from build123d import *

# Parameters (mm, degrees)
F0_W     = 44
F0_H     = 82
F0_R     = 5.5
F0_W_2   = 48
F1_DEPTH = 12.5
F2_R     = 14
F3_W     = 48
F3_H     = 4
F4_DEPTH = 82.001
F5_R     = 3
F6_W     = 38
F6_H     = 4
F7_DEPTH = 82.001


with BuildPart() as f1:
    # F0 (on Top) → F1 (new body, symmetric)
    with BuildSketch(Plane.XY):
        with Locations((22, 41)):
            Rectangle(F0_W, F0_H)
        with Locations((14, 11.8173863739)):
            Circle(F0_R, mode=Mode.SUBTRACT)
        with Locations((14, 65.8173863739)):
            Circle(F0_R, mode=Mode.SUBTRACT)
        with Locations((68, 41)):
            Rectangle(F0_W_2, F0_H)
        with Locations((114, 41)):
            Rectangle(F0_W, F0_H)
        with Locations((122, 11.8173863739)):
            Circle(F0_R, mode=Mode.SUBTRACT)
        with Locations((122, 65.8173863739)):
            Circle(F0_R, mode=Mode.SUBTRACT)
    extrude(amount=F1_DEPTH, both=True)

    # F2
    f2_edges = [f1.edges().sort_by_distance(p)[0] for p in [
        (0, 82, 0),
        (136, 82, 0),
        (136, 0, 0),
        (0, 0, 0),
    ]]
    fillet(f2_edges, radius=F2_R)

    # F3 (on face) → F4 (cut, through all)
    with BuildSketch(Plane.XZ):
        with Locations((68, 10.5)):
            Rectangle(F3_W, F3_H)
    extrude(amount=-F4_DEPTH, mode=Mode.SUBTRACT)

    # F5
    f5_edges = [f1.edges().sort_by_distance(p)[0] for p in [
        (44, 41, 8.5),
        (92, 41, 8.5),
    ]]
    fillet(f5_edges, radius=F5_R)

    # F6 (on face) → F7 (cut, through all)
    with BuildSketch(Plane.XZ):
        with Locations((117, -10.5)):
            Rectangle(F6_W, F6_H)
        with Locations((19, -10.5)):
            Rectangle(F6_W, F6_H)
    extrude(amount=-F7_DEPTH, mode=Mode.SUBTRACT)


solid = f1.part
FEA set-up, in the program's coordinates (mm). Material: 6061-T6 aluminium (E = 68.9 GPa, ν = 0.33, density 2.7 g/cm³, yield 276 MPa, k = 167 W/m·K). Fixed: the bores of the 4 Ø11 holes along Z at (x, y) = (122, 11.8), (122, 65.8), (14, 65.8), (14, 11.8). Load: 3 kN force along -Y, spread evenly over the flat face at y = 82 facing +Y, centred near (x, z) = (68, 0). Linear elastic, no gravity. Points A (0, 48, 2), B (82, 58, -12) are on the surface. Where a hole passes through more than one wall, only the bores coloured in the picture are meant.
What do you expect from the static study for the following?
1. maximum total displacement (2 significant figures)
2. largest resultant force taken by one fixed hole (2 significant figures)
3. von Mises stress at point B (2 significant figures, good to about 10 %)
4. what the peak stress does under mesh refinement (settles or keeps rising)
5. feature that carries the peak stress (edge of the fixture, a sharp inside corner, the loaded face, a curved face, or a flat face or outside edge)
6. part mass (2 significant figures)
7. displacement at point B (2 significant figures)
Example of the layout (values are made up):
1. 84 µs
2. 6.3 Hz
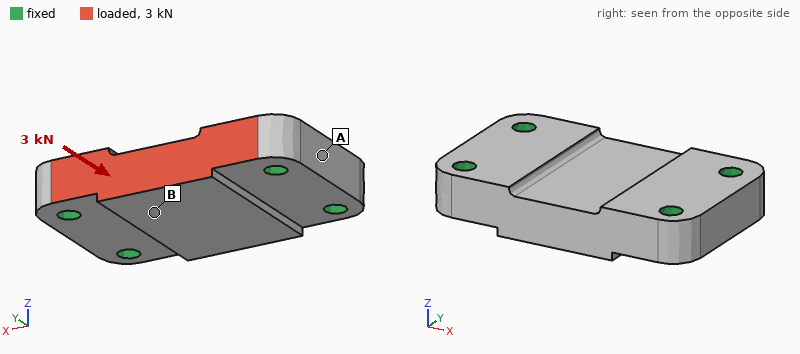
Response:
1. 2.0 µm
2. 990 N
3. 1.2 MPa
4. keeps rising
5. edge of the fixture
6. 610 g
7. 1.4 µm
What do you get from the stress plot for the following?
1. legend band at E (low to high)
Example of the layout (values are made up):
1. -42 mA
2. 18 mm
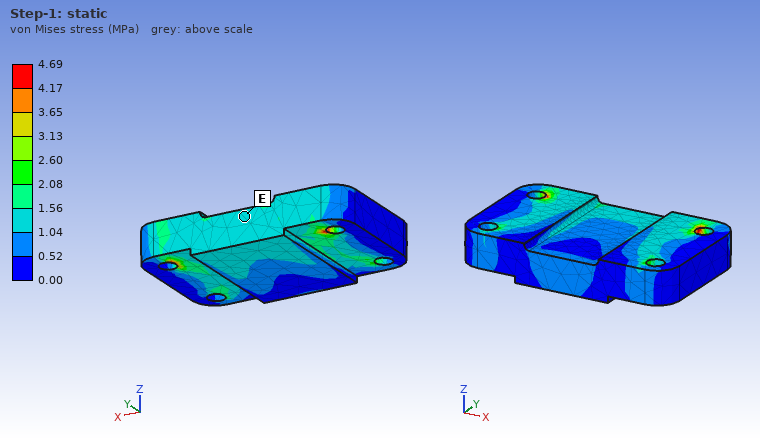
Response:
1. 1.04 to 1.56 MPa
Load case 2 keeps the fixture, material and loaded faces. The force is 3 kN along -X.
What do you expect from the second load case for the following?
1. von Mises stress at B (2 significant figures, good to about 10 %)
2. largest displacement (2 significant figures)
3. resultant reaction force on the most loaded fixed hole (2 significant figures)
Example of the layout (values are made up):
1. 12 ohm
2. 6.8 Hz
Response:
1. 0.65 MPa
2. 1.5 µm
3. 1.4 kN
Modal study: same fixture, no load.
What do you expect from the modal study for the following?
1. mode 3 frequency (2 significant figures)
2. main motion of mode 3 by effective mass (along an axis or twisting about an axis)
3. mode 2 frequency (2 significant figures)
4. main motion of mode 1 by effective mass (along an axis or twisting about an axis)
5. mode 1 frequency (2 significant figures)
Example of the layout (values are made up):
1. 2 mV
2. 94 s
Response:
1. 13 kHz
2. along Y
3. 9700 Hz
4. along Z
5. 7600 Hz
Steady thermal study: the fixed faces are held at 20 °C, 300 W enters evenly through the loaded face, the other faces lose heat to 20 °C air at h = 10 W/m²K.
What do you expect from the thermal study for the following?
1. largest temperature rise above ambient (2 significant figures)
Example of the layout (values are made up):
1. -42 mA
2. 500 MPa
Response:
1. 32 K
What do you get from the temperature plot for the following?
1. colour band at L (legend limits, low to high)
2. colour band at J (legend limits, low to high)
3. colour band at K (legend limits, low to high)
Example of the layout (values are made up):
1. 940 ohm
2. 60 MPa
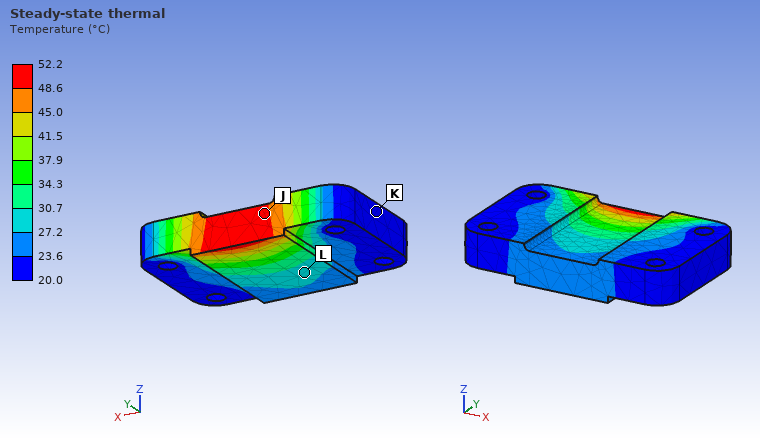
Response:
1. 27.2 to 30.7 °C
2. 48.6 to 52.2 °C
3. 20.0 to 23.6 °C
